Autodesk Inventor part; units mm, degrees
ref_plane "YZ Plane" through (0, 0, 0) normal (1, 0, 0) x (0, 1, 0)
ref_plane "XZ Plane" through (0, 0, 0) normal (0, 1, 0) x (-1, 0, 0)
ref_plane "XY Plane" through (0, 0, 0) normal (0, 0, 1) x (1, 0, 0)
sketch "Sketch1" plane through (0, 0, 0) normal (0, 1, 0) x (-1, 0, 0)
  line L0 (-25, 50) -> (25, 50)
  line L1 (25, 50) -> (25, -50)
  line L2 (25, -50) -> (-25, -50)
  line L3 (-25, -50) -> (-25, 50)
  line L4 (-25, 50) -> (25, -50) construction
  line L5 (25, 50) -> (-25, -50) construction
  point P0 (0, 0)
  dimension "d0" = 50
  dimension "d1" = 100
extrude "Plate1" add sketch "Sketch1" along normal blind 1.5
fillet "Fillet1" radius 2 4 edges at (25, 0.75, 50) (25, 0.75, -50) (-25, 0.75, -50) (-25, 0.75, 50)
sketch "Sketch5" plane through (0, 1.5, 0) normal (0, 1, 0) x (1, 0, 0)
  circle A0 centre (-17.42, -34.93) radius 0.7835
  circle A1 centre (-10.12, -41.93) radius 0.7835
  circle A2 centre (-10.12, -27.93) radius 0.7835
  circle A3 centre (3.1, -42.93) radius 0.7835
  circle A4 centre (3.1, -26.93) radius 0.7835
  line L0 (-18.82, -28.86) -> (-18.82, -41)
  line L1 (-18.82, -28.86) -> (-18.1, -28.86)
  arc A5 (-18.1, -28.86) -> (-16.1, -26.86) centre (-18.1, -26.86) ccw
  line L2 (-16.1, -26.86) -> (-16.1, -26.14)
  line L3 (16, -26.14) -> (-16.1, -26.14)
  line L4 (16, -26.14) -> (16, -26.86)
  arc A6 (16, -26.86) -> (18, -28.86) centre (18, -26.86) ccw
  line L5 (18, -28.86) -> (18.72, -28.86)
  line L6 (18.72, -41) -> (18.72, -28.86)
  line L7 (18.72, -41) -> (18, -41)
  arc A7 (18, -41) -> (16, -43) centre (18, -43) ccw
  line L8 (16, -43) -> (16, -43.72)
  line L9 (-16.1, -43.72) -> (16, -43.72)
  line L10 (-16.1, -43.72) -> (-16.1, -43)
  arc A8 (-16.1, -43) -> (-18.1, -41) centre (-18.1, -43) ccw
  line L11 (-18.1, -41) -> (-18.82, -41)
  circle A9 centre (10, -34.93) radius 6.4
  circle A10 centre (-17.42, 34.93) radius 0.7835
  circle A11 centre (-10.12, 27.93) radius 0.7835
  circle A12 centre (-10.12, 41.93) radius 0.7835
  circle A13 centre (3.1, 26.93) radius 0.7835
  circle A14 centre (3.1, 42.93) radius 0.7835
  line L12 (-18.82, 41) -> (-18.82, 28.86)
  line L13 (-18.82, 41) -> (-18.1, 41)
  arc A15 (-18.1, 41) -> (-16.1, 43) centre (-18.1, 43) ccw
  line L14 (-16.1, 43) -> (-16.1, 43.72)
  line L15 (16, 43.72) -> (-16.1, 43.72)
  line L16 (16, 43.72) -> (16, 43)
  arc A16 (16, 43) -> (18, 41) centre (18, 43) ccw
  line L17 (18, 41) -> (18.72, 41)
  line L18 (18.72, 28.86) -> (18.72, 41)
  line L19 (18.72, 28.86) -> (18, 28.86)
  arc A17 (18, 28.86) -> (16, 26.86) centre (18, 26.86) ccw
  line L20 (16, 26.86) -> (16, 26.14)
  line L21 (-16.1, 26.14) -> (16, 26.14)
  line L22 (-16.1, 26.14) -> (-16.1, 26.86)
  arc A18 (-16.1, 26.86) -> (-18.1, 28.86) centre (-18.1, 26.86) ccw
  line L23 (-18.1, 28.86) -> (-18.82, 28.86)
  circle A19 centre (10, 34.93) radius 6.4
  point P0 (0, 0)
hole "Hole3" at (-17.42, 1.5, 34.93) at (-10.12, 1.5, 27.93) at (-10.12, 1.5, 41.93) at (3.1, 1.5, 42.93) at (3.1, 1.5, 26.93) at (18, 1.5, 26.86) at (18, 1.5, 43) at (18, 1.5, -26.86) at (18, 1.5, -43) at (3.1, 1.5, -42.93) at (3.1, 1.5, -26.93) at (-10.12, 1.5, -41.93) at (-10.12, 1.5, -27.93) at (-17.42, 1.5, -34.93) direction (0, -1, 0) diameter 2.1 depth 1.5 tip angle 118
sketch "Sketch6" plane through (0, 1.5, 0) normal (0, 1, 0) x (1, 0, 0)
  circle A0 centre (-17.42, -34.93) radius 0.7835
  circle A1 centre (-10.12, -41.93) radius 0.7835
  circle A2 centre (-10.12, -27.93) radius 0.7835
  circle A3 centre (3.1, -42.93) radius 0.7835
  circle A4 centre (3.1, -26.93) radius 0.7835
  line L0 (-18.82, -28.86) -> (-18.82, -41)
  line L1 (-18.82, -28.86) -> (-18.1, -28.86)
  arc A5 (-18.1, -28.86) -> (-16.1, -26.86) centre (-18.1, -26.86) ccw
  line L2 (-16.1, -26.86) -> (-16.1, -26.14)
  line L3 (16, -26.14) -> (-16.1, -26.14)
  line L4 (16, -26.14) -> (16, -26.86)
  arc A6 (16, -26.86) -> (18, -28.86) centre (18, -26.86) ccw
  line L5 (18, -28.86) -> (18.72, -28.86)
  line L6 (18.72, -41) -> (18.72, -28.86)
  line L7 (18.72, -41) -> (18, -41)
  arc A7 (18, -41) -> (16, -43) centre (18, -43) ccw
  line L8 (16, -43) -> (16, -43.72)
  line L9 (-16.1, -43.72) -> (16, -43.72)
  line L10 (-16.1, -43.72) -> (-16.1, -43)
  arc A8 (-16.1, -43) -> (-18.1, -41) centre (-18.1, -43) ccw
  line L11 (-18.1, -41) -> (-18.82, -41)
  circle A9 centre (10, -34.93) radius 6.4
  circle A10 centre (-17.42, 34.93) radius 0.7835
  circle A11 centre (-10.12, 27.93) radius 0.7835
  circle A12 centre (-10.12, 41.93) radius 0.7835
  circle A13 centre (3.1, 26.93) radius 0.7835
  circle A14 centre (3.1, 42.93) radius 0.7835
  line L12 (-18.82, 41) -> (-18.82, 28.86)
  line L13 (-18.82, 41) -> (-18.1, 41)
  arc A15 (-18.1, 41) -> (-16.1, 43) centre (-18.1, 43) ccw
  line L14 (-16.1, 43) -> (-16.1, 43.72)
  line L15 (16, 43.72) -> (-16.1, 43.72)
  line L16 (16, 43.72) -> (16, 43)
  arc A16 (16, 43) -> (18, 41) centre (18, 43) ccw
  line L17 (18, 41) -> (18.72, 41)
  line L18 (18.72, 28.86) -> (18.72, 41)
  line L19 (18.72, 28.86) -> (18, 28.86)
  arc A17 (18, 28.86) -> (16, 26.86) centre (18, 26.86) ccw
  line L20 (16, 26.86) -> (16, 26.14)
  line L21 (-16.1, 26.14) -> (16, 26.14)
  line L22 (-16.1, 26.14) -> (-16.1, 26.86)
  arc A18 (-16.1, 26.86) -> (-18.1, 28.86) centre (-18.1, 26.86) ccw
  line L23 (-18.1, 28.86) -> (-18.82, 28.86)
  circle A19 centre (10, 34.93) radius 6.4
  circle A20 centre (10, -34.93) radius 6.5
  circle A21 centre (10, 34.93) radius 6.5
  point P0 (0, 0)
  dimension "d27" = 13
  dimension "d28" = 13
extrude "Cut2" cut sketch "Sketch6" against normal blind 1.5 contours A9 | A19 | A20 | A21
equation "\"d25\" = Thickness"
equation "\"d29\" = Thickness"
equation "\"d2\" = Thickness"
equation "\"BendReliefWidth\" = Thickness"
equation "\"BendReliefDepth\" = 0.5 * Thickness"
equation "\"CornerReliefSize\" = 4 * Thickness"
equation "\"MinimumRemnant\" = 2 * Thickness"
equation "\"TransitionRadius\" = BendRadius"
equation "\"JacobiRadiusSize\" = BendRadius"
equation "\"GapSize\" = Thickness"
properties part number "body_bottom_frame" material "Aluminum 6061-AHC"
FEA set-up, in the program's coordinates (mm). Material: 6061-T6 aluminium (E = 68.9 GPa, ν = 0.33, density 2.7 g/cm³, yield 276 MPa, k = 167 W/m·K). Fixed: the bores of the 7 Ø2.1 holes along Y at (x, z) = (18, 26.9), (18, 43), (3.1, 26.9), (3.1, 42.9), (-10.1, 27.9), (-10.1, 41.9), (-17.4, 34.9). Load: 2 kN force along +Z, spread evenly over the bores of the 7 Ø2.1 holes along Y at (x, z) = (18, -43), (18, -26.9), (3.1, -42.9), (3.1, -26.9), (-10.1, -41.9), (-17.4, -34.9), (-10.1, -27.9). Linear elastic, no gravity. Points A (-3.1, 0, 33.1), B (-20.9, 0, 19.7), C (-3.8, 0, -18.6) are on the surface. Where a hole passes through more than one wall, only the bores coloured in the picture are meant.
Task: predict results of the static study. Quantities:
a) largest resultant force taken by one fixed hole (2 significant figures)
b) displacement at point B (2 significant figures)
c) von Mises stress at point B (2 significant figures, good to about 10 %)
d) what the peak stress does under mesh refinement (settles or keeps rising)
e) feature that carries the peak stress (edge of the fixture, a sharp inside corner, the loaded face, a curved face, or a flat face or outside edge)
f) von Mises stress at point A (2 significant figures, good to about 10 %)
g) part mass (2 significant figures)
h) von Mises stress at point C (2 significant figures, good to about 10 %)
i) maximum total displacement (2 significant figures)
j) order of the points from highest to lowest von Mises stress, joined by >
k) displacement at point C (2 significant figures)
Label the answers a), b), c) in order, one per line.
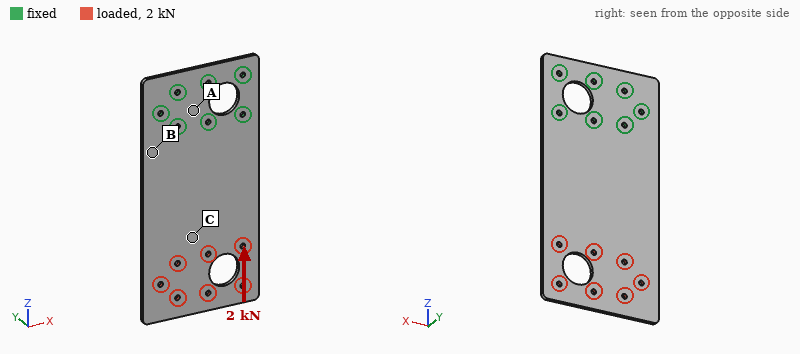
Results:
a) 550 N
b) 6.7 µm
c) 21 MPa
d) keeps rising
e) edge of the fixture
f) 8.1 MPa
g) 19 g
h) 32 MPa
i) 33 µm
j) C > B > A
k) 20 µm
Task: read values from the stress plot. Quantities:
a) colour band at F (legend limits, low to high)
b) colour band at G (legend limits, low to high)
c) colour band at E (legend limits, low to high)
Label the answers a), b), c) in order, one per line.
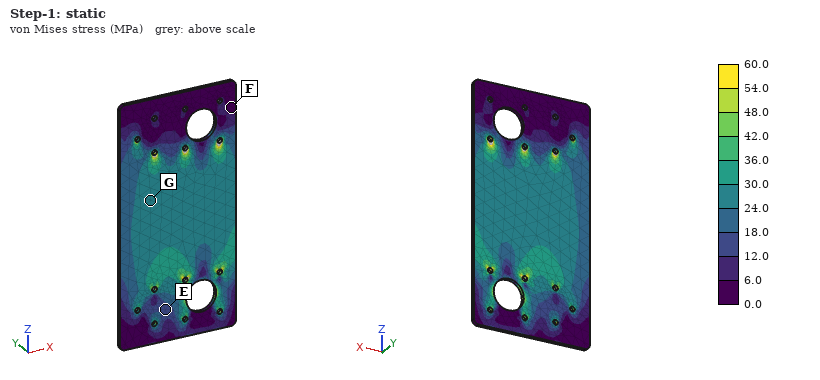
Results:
a) 0.0 to 6.0 MPa
b) 24.0 to 30.0 MPa
c) 12.0 to 18.0 MPa
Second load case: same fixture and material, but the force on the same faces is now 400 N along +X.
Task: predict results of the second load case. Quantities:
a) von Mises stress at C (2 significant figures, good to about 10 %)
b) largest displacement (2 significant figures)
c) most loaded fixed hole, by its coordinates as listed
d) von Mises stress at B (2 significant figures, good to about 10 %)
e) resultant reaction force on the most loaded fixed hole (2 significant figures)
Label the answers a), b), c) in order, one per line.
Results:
a) 12 MPa
b) 74 µm
c) (18, 26.9)
d) 26 MPa
e) 600 N
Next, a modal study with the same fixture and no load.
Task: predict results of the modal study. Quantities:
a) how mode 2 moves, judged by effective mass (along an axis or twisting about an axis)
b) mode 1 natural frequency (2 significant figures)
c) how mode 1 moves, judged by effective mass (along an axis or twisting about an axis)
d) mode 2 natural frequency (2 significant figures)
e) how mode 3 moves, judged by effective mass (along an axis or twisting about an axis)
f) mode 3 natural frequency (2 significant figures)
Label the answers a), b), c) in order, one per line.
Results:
a) twisting about Z
b) 220 Hz
c) along Y
d) 700 Hz
e) along Y
f) 1300 Hz
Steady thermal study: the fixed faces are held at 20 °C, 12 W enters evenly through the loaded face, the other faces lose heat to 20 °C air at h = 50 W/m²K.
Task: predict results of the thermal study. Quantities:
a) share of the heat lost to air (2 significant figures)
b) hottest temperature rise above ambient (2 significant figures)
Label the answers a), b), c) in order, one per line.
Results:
a) 59 %
b) 36 K
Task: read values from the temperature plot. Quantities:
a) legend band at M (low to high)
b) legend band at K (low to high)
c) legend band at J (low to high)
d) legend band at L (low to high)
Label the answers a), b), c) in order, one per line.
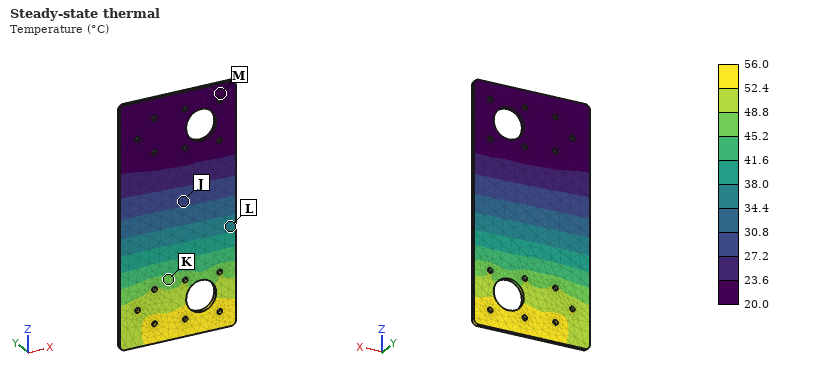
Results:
a) 20.0 to 23.6 °C
b) 45.2 to 48.8 °C
c) 27.2 to 30.8 °C
d) 34.4 to 38.0 °C
